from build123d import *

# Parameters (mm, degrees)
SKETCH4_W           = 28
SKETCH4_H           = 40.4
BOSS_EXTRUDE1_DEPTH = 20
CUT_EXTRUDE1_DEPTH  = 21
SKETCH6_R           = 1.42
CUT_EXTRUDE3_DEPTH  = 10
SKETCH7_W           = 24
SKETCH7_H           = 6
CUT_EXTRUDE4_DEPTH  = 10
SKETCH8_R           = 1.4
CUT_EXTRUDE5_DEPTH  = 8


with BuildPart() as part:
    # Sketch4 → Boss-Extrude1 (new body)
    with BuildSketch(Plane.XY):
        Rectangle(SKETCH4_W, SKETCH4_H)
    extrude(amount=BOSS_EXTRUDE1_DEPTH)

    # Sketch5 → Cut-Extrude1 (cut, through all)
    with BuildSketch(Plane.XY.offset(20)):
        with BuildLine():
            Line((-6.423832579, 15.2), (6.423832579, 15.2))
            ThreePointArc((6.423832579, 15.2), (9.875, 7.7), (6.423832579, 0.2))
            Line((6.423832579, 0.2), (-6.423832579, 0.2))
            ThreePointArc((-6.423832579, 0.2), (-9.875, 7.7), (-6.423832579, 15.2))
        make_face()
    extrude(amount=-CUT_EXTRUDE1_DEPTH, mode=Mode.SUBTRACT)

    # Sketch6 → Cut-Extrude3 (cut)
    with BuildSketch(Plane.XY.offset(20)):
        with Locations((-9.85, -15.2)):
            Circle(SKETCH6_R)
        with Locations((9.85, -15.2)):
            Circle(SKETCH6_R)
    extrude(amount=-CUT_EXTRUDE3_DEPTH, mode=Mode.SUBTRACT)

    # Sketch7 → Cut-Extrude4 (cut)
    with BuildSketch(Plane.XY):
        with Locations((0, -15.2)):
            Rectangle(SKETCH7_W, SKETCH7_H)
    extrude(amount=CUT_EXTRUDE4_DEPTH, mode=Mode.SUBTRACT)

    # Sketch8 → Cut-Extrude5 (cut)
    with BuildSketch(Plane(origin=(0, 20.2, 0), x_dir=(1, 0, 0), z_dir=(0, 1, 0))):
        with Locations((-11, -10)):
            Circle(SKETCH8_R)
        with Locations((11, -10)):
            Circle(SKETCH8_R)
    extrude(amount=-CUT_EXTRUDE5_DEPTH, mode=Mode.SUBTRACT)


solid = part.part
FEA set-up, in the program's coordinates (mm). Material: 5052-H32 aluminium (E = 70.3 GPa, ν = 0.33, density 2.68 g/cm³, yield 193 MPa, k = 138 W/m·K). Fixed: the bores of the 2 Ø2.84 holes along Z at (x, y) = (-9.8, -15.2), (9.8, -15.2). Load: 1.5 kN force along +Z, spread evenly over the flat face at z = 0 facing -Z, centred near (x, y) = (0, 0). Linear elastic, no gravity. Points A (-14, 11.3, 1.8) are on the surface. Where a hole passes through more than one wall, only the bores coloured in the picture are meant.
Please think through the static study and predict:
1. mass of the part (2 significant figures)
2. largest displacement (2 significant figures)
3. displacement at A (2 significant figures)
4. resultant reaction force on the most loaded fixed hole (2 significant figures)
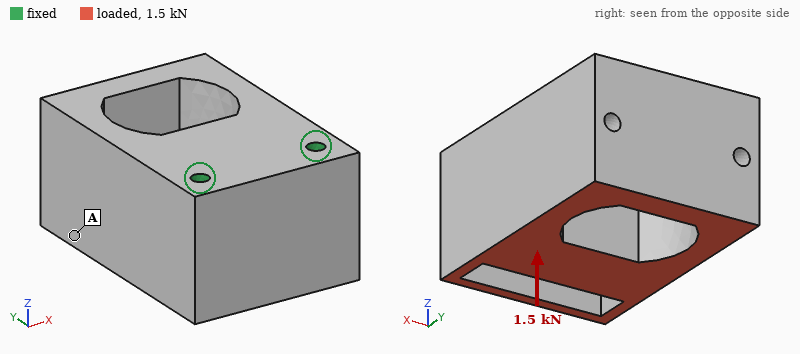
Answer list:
42 g
44 µm
32 µm
750 N
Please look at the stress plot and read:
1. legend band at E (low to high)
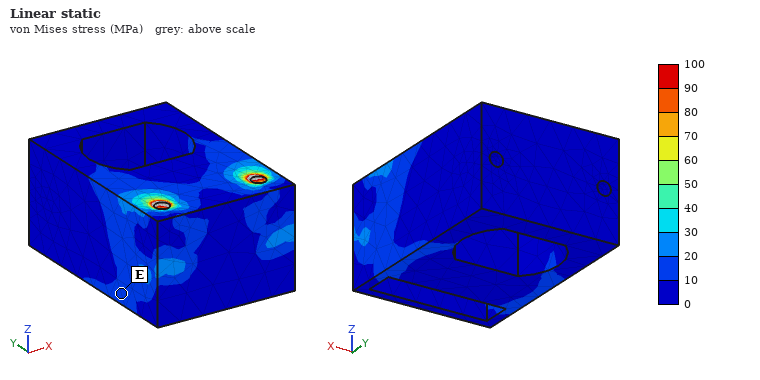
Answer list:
10 to 20 MPa
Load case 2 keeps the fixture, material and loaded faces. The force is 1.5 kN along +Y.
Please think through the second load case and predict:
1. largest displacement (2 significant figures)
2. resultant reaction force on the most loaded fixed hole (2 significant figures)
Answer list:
44 µm
750 N
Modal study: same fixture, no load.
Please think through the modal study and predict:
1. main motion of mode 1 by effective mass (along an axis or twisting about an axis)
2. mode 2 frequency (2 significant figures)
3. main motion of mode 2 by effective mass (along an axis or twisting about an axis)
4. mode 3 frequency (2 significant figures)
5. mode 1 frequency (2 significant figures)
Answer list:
along Z
8700 Hz
along X
13 kHz
5700 Hz
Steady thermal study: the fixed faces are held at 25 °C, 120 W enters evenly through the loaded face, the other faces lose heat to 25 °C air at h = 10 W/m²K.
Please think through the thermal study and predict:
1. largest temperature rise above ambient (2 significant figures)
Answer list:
66 K
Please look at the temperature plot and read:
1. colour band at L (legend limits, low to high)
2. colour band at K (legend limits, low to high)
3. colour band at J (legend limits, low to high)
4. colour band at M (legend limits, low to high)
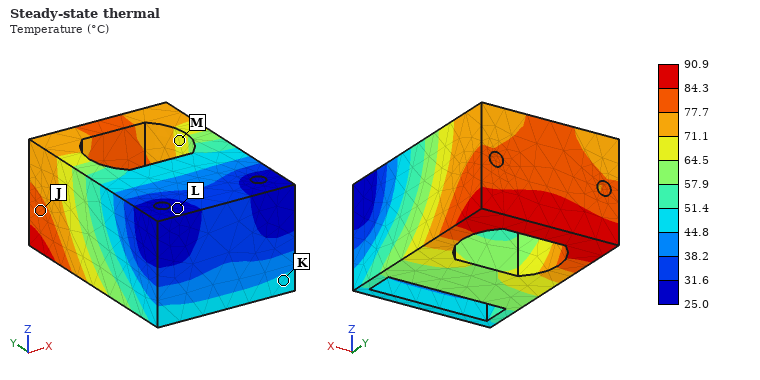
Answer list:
25.0 to 31.6 °C
44.8 to 51.4 °C
77.7 to 84.3 °C
64.5 to 71.1 °C
